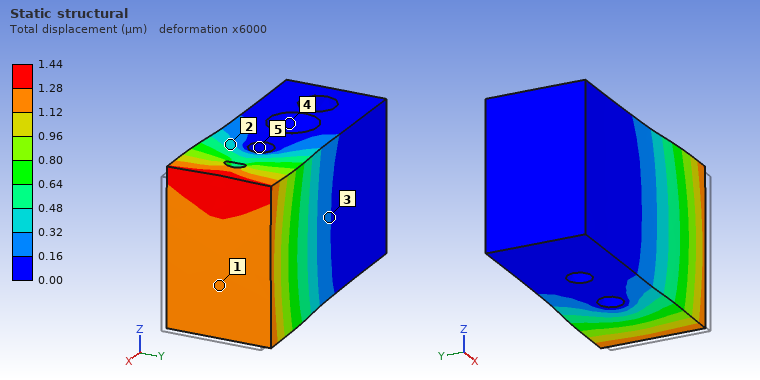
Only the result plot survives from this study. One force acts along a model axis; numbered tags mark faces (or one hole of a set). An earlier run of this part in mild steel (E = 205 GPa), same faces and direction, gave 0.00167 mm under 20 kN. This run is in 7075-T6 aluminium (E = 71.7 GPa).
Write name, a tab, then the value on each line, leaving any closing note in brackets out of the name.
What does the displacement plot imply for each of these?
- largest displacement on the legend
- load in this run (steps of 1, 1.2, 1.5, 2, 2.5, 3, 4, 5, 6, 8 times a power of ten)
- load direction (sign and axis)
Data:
largest displacement on the legend	1.44 µm
load in this run	6 kN
load direction	-X
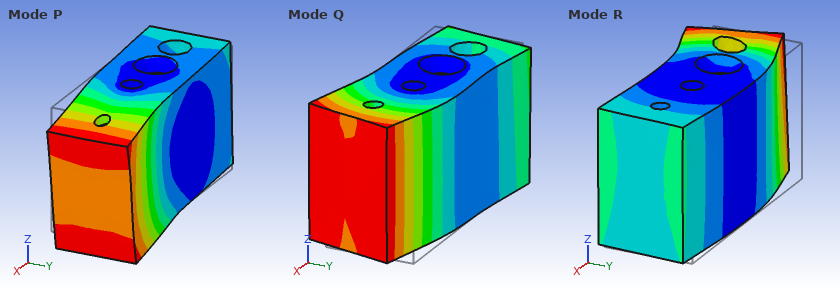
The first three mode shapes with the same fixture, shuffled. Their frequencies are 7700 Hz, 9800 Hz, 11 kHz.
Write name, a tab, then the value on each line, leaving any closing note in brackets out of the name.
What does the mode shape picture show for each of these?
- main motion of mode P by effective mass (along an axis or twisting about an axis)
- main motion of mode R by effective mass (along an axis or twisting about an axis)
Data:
main motion of mode P by effective mass	along Z
main motion of mode R by effective mass	along Y
